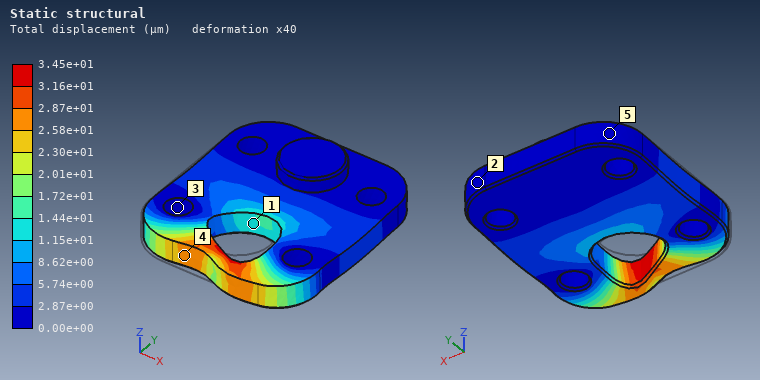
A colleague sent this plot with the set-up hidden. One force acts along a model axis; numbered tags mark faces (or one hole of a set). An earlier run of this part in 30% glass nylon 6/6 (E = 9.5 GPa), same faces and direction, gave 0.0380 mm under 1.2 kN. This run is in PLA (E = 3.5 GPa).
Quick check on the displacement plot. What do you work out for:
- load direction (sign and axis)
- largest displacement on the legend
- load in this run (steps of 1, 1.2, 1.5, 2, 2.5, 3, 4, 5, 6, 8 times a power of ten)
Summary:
+X
3.45e+01 µm
400 N
